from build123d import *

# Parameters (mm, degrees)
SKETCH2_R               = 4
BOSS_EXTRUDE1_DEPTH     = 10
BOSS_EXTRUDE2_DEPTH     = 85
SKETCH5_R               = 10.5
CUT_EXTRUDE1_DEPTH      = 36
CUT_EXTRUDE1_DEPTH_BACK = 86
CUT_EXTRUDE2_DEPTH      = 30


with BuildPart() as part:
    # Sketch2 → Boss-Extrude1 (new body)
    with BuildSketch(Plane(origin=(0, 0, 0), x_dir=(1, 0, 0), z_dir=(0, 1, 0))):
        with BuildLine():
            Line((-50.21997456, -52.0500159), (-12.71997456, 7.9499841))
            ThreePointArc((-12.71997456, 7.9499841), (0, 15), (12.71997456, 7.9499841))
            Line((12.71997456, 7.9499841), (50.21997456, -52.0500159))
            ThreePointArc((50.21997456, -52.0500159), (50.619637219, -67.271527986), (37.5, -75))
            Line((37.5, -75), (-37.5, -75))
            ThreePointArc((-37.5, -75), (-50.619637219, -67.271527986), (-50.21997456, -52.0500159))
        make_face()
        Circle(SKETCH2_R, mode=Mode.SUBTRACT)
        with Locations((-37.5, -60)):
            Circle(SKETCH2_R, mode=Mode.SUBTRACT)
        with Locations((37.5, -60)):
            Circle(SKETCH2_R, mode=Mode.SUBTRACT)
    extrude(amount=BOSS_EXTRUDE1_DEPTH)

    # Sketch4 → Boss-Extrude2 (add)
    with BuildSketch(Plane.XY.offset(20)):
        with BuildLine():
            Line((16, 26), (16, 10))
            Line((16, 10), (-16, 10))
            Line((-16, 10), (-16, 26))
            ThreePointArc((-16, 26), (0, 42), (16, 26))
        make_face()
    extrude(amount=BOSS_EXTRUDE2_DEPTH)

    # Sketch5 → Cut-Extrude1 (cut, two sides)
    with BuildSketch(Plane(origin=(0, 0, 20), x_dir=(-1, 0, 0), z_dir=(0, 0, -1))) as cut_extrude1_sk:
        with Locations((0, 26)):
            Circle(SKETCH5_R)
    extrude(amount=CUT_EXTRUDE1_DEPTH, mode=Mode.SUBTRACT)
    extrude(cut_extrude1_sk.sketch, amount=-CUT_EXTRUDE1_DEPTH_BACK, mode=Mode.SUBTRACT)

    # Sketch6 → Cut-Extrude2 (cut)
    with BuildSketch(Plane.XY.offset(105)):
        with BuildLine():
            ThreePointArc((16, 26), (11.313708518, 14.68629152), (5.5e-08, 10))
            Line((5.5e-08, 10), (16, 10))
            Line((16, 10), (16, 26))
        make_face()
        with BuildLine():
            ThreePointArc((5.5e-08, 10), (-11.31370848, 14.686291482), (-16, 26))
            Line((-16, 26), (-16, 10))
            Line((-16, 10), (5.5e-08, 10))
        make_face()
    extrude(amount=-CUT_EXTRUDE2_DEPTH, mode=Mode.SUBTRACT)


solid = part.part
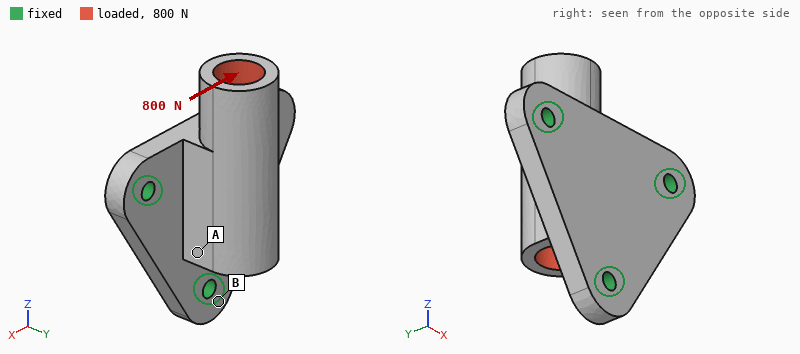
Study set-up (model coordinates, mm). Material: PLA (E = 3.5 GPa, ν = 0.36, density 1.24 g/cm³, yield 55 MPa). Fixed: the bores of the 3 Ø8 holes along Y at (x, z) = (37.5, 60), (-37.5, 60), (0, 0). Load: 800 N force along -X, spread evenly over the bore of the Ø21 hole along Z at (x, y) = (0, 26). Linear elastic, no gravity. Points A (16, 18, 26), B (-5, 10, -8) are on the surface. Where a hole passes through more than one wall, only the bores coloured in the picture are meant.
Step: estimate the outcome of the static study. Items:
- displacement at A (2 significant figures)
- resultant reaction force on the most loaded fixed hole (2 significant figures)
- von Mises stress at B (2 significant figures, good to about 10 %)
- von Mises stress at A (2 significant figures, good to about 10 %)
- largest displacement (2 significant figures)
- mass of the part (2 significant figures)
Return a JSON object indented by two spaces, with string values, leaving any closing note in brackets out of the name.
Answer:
{
  "displacement at A": "0.044 mm",
  "resultant reaction force on the most loaded fixed hole": "460 N",
  "von Mises stress at B": "0.62 MPa",
  "von Mises stress at A": "2.2 MPa",
  "largest displacement": "0.17 mm",
  "mass of the part": "130 g"
}
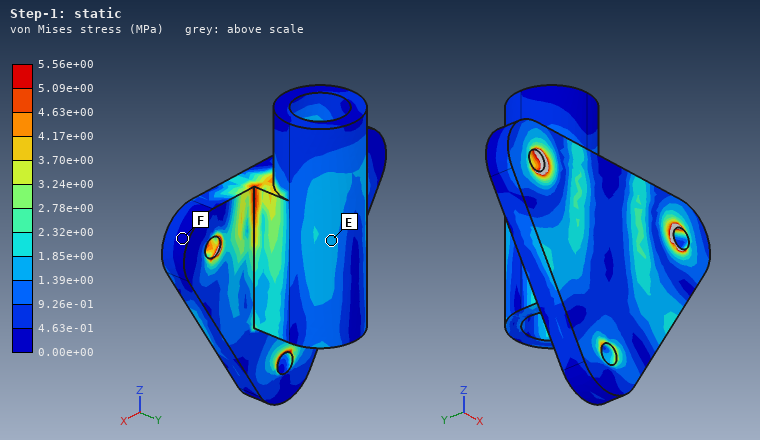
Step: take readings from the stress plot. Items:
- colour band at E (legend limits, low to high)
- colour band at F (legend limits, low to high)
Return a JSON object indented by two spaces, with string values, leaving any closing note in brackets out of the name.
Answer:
{
  "colour band at E": "1.39e+00 to 1.85e+00 MPa",
  "colour band at F": "0.00e+00 to 4.63e-01 MPa"
}
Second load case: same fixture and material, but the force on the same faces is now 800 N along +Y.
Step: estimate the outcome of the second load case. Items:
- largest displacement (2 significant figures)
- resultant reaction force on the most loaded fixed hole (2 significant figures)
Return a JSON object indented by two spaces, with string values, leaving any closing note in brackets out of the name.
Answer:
{
  "largest displacement": "0.25 mm",
  "resultant reaction force on the most loaded fixed hole": "420 N"
}
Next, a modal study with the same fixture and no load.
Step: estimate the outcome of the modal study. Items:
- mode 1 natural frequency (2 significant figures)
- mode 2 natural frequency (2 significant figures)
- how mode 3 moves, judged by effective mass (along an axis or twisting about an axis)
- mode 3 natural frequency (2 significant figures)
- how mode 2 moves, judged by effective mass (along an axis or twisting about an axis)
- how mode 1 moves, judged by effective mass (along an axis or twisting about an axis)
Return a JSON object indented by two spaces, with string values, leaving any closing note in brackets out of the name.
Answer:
{
  "mode 1 natural frequency": "1400 Hz",
  "mode 2 natural frequency": "1900 Hz",
  "how mode 3 moves, judged by effective mass": "along Y",
  "mode 3 natural frequency": "2300 Hz",
  "how mode 2 moves, judged by effective mass": "along X",
  "how mode 1 moves, judged by effective mass": "along Y"
}
